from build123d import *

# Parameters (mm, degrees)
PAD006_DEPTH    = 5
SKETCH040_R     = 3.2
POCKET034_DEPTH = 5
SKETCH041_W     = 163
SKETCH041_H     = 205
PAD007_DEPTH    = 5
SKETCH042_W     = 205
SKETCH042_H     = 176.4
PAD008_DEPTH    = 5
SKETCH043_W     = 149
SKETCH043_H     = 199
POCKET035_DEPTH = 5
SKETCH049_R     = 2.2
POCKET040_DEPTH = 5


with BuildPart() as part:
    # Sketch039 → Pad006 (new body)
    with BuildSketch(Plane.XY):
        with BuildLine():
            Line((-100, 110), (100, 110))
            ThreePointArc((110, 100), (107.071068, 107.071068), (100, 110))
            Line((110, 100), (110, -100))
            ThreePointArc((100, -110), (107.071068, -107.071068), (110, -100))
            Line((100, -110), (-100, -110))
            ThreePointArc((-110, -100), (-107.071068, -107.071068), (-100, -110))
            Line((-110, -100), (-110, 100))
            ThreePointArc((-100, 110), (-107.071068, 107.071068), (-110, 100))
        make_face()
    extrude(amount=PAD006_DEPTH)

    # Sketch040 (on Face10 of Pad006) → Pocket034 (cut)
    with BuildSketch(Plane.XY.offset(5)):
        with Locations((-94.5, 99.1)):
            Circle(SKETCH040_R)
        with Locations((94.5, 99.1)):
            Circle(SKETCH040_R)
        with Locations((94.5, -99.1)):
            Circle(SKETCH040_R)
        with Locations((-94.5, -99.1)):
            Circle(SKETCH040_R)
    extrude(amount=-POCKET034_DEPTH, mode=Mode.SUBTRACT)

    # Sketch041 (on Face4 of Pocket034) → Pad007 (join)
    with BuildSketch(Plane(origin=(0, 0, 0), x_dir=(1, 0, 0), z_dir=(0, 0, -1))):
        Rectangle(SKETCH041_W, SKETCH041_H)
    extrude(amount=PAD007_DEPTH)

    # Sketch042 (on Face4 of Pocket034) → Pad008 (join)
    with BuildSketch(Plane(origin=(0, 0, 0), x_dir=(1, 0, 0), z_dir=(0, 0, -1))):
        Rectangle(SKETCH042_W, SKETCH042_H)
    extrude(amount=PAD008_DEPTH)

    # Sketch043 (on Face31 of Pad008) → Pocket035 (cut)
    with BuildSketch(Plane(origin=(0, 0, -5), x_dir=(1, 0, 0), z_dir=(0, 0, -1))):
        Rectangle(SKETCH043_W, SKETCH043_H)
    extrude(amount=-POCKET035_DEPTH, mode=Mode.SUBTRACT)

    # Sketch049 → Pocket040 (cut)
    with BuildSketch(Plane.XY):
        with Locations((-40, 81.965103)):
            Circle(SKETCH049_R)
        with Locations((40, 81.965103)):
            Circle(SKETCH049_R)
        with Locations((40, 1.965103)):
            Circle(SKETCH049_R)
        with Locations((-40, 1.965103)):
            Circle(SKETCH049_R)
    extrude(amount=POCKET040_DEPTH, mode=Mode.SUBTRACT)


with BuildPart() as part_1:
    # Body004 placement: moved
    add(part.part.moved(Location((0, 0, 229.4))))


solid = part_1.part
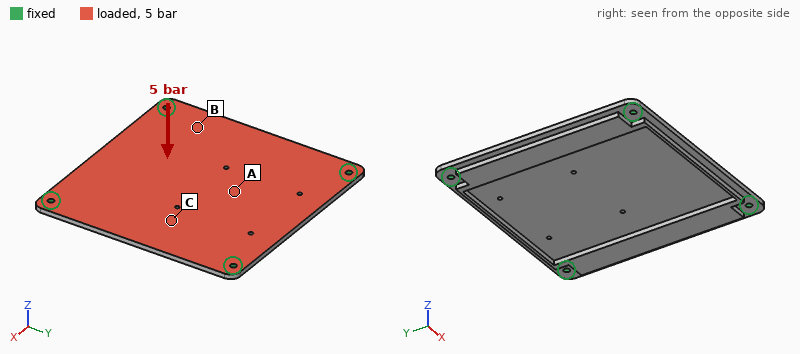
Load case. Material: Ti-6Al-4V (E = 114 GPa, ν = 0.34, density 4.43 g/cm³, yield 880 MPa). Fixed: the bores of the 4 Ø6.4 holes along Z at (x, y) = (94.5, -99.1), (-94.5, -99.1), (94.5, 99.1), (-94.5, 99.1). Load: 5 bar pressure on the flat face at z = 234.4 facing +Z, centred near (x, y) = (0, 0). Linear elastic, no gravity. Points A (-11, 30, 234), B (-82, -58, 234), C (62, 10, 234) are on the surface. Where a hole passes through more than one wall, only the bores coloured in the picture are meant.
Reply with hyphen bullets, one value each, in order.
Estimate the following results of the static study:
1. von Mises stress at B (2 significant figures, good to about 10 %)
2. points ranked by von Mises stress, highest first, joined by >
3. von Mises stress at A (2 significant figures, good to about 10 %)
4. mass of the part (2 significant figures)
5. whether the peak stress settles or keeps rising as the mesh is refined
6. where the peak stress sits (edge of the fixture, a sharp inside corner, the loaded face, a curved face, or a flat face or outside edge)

- 66 MPa
- A > C > B
- 200 MPa
- 1.3 kg
- keeps rising
- edge of the fixture
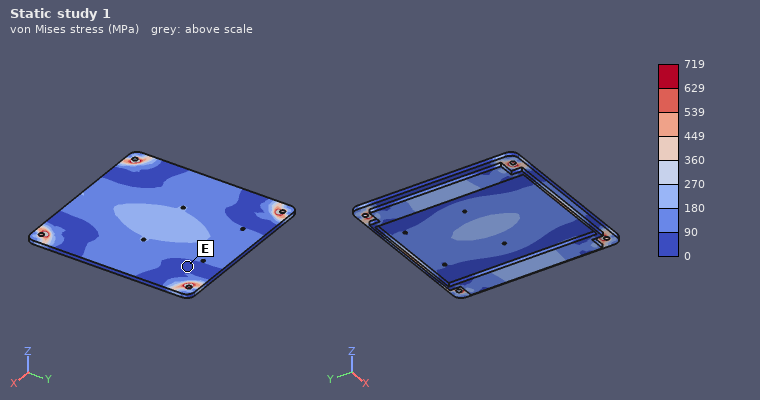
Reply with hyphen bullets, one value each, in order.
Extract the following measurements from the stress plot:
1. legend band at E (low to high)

- 0 to 90 MPa
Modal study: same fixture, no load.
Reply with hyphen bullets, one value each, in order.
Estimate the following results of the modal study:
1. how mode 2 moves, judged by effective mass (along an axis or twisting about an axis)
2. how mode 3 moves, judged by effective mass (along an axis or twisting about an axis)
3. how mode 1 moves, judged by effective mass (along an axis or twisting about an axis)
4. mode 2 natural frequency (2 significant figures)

- twisting about Y
- twisting about X
- along Z
- 930 Hz
